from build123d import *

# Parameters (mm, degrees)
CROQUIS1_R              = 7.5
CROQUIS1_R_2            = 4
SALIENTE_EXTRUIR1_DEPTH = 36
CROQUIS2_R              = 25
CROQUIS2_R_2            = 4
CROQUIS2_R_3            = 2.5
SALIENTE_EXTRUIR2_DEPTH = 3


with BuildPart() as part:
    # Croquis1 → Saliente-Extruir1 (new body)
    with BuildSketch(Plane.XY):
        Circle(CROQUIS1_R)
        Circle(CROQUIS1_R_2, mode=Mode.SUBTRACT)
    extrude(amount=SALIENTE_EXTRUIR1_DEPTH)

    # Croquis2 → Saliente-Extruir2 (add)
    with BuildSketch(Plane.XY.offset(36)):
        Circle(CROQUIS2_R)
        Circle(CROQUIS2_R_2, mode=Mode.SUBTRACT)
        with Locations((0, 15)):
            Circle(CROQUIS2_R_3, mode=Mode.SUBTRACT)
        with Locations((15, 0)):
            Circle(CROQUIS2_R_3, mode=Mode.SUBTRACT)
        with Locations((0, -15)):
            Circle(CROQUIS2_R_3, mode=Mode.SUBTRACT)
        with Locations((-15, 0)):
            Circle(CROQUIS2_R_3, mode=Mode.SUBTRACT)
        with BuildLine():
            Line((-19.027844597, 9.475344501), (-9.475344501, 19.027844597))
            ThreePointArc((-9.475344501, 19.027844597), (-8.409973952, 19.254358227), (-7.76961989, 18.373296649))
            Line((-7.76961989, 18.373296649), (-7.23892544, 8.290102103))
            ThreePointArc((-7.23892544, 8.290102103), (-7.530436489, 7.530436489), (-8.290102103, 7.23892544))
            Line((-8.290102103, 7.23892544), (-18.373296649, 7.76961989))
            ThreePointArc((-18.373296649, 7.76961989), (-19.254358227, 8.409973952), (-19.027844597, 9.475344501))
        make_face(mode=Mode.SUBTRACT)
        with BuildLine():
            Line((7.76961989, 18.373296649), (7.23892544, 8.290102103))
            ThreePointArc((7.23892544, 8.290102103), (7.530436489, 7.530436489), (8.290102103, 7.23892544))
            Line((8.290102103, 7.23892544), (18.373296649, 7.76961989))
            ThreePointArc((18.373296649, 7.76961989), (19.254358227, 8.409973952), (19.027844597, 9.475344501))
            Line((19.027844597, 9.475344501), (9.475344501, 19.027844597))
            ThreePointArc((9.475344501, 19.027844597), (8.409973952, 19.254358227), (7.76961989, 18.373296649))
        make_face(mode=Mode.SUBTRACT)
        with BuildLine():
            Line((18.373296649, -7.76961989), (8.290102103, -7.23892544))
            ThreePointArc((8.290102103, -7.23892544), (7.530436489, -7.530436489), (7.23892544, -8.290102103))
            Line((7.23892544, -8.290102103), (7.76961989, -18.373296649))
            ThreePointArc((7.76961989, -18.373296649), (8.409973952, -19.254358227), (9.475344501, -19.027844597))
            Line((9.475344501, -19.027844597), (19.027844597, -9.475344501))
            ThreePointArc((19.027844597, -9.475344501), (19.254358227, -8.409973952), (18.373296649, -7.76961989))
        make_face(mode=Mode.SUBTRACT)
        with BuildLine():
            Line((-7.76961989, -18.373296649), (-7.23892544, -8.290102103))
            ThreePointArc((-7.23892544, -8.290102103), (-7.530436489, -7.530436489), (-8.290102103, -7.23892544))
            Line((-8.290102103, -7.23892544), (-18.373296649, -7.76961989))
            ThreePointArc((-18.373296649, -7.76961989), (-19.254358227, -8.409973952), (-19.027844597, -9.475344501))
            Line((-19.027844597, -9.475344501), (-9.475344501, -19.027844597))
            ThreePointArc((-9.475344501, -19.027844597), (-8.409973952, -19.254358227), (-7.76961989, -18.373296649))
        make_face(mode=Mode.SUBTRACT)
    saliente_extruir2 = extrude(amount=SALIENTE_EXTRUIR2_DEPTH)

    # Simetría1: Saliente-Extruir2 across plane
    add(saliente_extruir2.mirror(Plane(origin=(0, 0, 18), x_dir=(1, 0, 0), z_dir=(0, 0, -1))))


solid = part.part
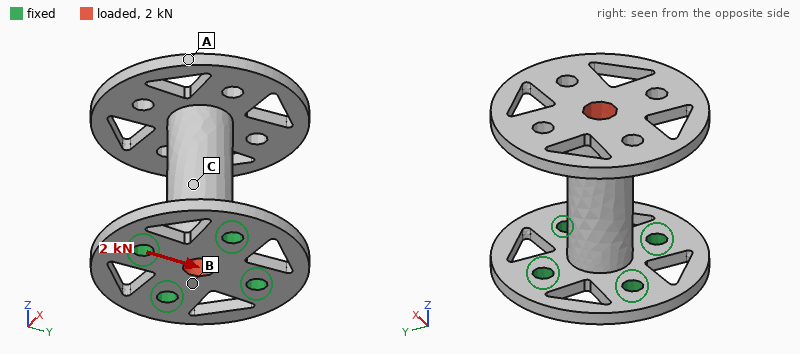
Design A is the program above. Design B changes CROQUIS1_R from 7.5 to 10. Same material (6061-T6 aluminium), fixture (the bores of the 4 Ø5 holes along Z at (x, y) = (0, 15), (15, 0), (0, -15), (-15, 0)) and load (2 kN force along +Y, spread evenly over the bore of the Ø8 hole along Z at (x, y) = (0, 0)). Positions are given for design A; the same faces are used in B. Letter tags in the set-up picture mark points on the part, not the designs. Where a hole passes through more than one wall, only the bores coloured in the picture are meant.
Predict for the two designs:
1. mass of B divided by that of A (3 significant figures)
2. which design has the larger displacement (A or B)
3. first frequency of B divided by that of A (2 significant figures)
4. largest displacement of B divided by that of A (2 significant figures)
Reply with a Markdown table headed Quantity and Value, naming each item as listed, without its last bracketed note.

| Quantity | Value |
|---|---|
| mass of B divided by that of A | 1.37 |
| which design has the larger displacement | A |
| first frequency of B divided by that of A | 1.6 |
| largest displacement of B divided by that of A | 0.33 |
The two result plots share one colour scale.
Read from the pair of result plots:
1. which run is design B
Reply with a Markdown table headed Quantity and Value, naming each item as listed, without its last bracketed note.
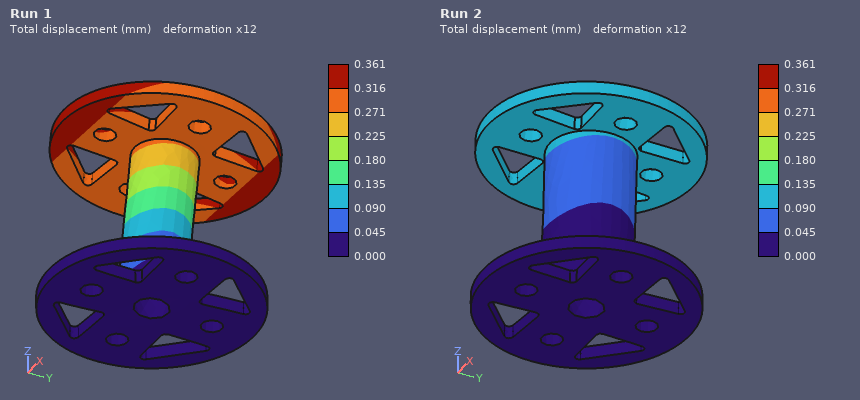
| Quantity | Value |
|---|---|
| which run is design B | Run 2 |
